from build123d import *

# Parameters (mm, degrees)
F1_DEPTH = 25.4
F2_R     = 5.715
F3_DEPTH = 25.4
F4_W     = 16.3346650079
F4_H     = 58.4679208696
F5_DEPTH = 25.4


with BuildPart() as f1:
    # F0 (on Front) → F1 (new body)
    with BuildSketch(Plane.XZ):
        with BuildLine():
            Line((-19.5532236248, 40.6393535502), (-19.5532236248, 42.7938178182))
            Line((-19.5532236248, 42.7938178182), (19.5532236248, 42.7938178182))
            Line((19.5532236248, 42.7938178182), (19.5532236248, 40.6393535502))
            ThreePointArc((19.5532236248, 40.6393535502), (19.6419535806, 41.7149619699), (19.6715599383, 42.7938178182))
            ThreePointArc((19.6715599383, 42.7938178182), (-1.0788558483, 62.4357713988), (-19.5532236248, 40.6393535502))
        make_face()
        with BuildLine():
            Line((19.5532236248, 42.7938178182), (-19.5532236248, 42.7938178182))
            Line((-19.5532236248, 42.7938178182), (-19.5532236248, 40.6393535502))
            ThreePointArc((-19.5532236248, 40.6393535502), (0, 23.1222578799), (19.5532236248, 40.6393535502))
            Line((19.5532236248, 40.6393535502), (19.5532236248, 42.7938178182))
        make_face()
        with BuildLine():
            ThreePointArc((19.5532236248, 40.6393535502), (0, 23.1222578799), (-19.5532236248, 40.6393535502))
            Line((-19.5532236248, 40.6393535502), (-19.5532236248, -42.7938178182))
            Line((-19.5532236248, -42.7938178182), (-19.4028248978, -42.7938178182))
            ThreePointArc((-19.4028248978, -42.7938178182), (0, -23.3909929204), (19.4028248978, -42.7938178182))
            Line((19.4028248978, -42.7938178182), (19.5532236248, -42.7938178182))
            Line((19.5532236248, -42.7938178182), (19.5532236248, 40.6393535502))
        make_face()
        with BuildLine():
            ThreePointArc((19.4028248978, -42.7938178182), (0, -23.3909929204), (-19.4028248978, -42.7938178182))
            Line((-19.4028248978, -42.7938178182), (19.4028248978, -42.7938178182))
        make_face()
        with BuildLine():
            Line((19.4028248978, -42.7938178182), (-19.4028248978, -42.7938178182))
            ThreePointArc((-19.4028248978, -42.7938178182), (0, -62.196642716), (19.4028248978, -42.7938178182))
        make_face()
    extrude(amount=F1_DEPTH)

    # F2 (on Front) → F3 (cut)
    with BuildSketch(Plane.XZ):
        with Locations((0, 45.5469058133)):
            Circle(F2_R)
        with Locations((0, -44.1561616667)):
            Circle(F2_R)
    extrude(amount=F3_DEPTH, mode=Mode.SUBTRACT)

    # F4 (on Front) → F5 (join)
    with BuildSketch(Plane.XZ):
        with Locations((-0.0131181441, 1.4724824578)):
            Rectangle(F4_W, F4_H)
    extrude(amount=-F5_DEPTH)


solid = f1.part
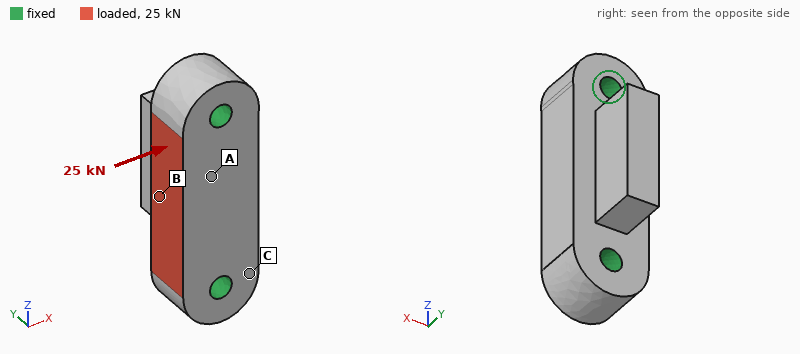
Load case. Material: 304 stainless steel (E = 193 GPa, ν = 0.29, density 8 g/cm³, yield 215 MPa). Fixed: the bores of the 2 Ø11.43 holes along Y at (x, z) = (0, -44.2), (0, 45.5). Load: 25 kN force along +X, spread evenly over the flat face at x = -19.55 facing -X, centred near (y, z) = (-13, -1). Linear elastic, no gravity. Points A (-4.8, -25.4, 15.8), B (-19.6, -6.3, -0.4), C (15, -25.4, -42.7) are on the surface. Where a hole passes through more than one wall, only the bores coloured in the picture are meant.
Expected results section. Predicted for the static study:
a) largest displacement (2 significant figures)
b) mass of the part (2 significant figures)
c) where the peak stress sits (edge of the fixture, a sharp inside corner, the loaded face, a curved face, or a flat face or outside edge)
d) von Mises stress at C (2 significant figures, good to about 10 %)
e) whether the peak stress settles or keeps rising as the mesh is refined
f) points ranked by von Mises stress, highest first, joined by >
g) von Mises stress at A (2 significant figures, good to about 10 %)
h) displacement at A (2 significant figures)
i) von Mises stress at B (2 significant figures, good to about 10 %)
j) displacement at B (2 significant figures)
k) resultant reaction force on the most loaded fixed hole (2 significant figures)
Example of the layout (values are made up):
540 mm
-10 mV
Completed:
9.0 µm
1.1 kg
edge of the fixture
6.4 MPa
keeps rising
B > A > C
14 MPa
7.3 µm
25 MPa
8.4 µm
13 kN
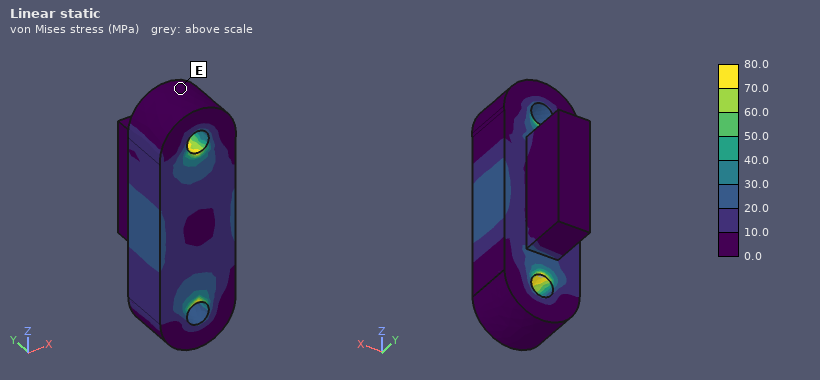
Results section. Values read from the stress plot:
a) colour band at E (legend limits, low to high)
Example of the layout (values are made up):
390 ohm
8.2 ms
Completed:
0.0 to 10.0 MPa
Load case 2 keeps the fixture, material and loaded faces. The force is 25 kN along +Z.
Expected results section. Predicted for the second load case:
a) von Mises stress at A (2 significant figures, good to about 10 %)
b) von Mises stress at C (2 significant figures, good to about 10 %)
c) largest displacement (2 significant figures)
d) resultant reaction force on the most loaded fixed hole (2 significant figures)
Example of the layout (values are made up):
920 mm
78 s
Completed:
13 MPa
4.4 MPa
3.9 µm
14 kN
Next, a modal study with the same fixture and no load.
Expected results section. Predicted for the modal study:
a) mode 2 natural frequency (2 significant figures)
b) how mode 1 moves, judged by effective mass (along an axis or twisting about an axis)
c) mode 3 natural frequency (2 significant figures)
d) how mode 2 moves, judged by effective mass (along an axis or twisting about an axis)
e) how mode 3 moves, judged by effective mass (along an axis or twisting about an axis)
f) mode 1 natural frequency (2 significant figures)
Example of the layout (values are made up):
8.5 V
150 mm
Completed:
11 kHz
along X
12 kHz
along Y
along X
7400 Hz
